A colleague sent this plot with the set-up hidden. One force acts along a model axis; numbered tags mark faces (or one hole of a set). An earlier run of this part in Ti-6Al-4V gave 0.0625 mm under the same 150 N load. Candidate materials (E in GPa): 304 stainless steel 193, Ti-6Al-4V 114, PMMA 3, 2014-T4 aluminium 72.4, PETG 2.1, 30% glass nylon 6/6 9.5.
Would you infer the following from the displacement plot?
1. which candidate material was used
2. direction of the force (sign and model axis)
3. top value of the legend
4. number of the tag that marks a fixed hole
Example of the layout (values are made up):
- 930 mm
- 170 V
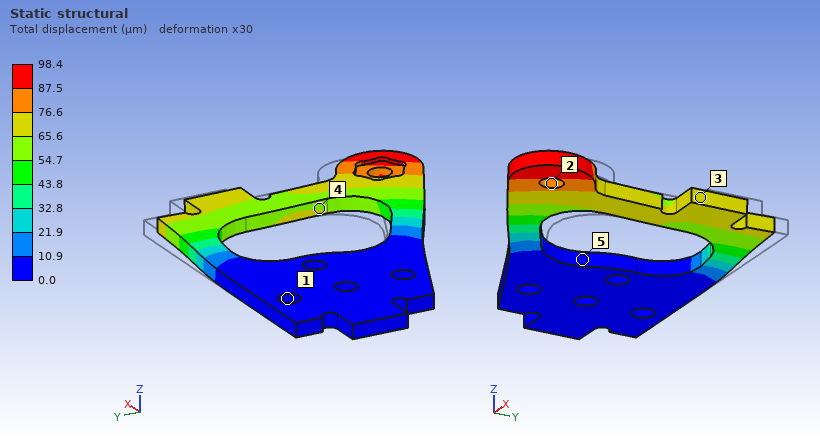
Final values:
- 2014-T4 aluminium
- -Y
- 98.4 µm
- 1
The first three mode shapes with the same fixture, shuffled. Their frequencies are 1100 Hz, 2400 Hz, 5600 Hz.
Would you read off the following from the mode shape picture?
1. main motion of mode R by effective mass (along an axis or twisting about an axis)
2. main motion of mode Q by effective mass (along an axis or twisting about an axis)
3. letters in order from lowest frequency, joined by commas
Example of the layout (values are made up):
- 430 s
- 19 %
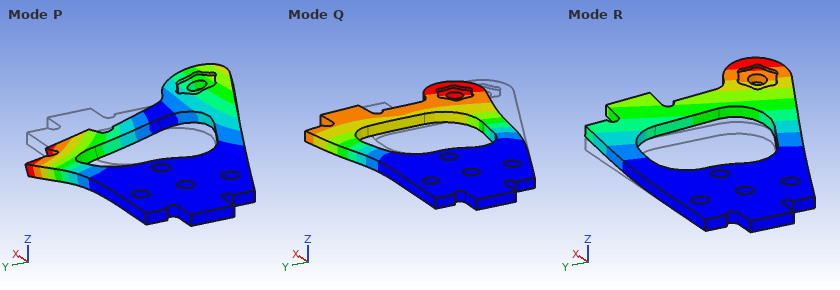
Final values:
- along Z
- along Y
- R, P, Q
